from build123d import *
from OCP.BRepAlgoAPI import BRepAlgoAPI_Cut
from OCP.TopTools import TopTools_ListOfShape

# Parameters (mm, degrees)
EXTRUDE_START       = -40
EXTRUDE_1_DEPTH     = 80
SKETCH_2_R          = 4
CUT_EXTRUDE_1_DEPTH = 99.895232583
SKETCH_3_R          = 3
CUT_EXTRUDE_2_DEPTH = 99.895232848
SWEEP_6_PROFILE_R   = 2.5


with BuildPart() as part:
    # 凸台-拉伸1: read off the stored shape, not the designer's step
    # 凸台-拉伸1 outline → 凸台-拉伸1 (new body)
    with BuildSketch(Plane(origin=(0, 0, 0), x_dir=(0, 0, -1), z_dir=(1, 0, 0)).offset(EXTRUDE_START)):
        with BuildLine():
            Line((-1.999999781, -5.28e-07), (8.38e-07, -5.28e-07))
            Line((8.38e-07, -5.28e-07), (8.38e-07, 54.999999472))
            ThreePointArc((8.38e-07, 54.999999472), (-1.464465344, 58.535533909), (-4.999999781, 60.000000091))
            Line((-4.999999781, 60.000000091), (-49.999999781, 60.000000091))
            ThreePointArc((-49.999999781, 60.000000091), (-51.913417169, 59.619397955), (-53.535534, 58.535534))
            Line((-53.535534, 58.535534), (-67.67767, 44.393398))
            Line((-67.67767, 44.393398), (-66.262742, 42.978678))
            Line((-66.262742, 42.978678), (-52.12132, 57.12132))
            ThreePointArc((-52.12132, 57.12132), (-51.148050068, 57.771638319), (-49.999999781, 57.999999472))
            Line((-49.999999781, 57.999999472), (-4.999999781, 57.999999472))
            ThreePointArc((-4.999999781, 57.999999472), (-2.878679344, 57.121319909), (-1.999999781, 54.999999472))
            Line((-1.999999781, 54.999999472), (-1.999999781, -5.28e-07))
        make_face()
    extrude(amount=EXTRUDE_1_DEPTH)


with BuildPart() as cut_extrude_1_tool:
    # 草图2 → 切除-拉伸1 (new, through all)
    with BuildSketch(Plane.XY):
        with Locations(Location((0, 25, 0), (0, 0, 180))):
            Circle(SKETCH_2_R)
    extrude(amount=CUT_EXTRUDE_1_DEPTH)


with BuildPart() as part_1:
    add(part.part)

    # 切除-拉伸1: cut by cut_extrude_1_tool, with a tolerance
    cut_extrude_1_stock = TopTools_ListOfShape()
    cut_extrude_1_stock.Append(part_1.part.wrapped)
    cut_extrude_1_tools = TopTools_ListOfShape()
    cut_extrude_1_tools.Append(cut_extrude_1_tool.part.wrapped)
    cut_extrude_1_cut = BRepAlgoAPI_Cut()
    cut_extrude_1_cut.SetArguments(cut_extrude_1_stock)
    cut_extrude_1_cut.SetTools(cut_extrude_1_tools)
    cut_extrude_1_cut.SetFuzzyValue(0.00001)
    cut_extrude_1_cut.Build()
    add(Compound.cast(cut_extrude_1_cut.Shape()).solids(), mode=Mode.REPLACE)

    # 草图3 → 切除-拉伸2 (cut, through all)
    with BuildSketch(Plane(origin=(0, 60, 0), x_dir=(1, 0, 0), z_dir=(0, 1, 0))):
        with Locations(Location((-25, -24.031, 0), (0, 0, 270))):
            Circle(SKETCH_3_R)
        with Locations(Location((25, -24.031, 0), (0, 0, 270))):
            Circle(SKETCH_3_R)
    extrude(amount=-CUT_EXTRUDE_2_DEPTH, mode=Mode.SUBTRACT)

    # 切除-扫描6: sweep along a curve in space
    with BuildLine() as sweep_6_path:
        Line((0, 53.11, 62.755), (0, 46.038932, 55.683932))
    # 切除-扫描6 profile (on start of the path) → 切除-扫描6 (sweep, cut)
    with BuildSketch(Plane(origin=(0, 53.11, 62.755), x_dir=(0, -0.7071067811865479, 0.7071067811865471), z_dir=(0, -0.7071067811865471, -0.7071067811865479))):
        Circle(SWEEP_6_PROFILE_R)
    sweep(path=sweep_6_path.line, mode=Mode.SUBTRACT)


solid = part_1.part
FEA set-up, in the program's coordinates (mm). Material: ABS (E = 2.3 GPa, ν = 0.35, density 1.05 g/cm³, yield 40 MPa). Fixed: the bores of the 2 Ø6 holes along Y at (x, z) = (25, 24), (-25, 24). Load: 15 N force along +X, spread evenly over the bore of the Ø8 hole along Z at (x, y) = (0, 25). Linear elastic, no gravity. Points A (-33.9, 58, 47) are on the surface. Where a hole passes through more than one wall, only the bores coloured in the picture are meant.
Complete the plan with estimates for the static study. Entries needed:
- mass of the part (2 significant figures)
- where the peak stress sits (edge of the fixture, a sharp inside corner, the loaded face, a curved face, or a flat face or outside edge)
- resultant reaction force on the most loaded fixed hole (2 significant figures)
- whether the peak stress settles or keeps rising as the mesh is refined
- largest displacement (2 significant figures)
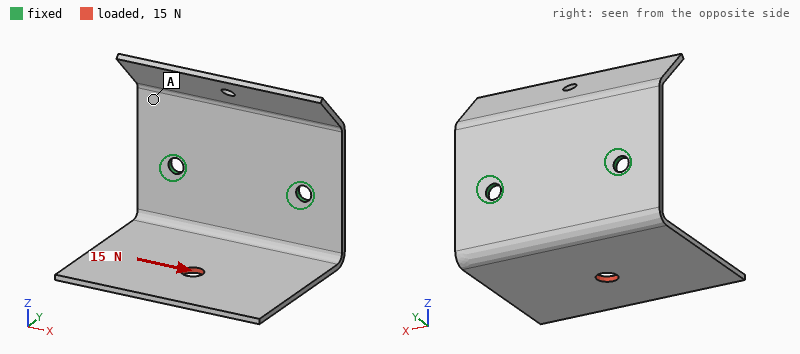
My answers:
21 g
edge of the fixture
14 N
keeps rising
1.1 mm
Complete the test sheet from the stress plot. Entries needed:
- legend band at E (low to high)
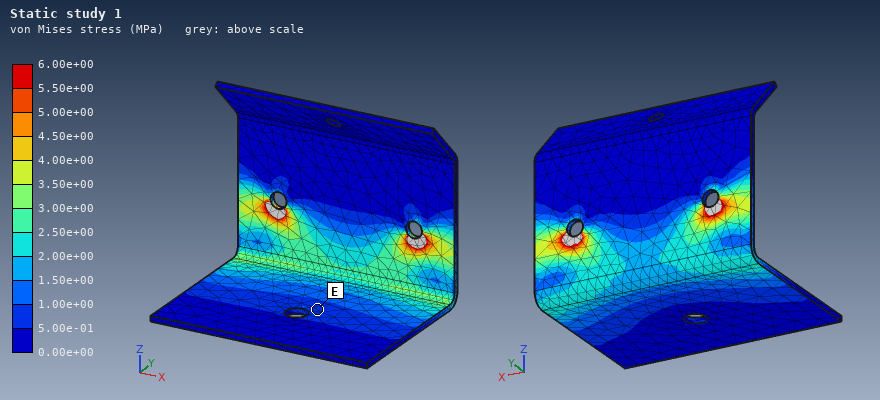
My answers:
5.00e-01 to 1.00e+00 MPa
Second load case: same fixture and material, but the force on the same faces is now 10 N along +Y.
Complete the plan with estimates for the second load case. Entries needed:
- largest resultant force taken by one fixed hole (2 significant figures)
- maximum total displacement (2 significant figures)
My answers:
5.0 N
1.2 mm
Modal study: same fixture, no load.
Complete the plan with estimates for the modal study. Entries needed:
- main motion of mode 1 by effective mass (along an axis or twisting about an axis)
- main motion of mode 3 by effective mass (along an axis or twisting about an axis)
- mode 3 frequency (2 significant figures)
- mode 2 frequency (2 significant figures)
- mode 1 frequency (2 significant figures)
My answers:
along Z
along Y
220 Hz
200 Hz
90 Hz
